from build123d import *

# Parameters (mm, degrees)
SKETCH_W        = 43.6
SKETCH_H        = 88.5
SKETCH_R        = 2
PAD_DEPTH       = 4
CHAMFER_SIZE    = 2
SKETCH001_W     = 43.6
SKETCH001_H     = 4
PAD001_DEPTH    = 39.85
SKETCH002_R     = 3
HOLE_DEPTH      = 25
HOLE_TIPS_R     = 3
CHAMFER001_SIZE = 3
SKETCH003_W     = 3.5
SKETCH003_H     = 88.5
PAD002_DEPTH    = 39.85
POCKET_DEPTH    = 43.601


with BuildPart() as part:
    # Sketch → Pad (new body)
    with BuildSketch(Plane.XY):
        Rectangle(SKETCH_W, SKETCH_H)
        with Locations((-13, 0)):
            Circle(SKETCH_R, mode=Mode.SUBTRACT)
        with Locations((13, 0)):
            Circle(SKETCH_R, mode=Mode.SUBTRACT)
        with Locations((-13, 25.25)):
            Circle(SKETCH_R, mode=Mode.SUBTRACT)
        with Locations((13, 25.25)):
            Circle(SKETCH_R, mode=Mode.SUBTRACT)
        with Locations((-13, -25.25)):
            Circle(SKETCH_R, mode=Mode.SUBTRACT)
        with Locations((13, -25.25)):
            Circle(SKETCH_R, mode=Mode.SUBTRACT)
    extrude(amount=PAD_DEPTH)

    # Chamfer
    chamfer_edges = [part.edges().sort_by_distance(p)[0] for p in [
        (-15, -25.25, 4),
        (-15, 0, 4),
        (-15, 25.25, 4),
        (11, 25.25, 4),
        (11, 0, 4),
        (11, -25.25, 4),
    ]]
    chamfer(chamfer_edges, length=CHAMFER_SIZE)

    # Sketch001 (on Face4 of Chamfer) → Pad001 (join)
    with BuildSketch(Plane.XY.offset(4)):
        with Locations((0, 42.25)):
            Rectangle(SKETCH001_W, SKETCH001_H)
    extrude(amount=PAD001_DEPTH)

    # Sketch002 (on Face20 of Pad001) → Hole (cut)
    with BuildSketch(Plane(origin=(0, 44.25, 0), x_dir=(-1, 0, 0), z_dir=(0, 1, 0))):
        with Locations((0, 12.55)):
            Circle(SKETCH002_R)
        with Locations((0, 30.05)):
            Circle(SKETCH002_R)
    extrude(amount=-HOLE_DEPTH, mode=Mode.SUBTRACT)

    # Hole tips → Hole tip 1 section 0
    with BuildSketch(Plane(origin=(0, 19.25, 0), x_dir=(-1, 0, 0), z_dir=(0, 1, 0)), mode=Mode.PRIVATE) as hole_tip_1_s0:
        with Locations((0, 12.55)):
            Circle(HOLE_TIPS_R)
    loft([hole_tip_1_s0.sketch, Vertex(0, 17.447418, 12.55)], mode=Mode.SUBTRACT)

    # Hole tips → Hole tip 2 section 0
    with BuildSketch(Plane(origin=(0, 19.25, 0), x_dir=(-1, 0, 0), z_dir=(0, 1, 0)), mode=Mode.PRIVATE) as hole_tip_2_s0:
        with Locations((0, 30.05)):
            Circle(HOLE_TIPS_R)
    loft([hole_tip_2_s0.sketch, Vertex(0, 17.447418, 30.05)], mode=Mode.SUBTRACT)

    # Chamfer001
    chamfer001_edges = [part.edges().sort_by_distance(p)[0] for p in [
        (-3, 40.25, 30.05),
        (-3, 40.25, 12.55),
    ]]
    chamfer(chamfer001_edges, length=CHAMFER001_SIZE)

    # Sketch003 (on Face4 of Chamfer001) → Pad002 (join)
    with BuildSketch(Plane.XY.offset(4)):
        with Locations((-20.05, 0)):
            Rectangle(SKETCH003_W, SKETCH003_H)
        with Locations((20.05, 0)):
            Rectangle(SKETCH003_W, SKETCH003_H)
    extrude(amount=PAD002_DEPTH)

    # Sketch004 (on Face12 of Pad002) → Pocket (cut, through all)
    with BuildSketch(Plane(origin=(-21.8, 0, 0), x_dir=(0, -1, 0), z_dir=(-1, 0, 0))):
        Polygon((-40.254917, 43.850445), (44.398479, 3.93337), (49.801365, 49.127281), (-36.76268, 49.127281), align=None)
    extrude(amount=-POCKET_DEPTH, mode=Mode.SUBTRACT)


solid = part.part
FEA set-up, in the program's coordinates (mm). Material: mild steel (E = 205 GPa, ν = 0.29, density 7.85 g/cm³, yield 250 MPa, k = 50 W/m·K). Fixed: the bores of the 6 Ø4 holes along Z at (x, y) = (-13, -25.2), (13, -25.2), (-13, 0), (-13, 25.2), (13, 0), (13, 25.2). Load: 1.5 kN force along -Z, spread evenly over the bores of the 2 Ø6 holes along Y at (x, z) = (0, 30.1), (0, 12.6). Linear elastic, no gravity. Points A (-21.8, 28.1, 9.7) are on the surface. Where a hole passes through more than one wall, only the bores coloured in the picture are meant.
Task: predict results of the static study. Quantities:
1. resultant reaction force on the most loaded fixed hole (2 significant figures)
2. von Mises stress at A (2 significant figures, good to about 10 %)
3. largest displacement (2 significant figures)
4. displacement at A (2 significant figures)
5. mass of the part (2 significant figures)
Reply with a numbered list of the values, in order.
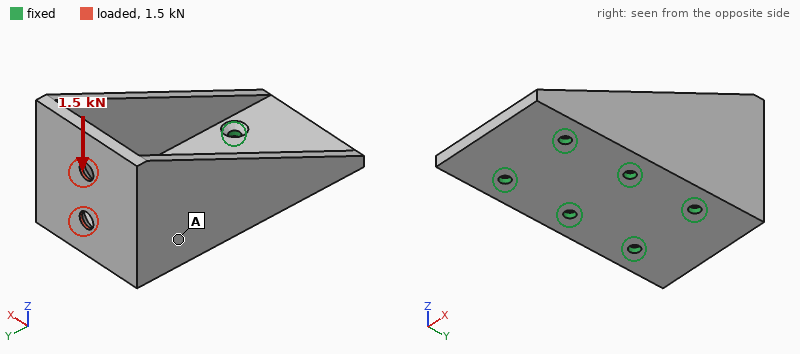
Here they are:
1. 1.1 kN
2. 14 MPa
3. 18 µm
4. 6.3 µm
5. 260 g
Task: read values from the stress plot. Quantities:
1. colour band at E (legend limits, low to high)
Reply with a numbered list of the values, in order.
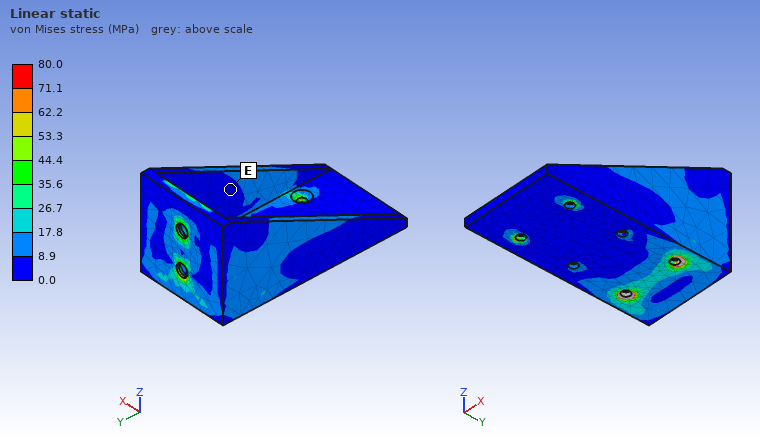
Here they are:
1. 0.0 to 8.9 MPa
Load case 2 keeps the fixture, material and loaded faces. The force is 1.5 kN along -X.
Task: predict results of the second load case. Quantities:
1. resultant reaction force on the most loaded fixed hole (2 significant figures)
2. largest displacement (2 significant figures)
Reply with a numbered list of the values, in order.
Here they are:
1. 1.6 kN
2. 39 µm
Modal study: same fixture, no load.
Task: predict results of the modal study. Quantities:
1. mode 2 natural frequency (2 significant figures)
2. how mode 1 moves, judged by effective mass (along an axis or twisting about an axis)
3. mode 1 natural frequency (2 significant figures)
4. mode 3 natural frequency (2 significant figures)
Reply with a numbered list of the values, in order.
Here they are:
1. 4700 Hz
2. along X
3. 3200 Hz
4. 5400 Hz
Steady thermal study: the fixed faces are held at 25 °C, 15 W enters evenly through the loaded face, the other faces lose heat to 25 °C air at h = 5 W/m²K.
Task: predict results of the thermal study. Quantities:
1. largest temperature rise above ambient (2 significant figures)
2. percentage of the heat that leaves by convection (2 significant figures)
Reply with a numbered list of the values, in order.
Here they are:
1. 48 K
2. 7.3 %
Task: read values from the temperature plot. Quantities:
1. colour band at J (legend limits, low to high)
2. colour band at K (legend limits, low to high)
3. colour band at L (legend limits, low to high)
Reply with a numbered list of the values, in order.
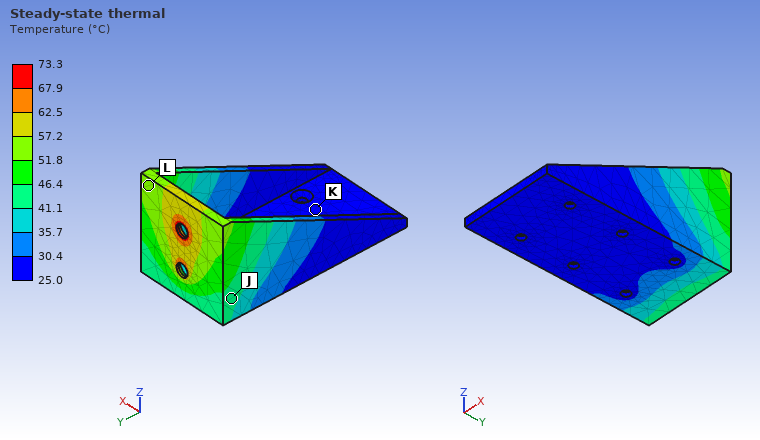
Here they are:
1. 41.1 to 46.4 °C
2. 25.0 to 30.4 °C
3. 51.8 to 57.2 °C
